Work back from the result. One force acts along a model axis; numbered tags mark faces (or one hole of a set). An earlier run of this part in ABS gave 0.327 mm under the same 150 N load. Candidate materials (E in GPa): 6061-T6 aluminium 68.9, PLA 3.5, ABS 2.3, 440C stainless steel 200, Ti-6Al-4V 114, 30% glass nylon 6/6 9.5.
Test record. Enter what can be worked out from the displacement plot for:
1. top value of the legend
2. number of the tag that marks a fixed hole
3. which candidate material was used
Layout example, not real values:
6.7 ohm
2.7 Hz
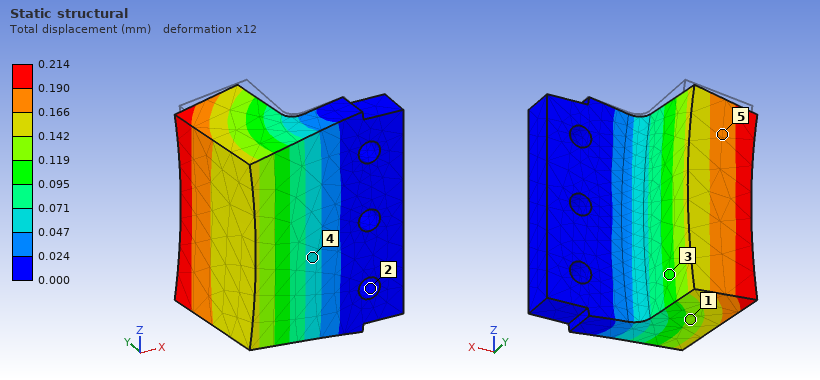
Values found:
0.214 mm
2
PLA
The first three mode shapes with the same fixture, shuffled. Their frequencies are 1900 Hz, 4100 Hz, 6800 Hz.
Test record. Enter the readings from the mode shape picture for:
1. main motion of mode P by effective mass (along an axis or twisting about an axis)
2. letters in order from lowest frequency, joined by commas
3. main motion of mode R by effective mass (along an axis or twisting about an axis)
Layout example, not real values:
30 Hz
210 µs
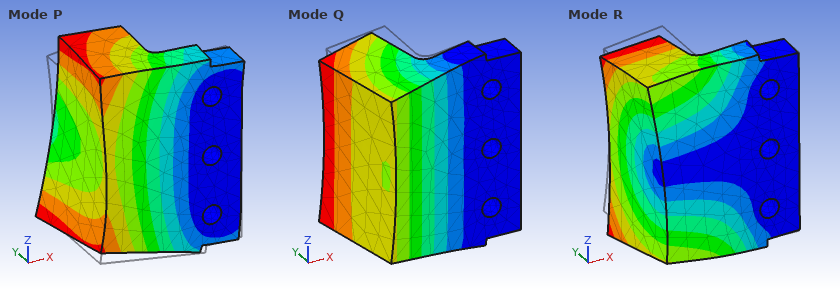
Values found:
along Z
Q, R, P
along Z
